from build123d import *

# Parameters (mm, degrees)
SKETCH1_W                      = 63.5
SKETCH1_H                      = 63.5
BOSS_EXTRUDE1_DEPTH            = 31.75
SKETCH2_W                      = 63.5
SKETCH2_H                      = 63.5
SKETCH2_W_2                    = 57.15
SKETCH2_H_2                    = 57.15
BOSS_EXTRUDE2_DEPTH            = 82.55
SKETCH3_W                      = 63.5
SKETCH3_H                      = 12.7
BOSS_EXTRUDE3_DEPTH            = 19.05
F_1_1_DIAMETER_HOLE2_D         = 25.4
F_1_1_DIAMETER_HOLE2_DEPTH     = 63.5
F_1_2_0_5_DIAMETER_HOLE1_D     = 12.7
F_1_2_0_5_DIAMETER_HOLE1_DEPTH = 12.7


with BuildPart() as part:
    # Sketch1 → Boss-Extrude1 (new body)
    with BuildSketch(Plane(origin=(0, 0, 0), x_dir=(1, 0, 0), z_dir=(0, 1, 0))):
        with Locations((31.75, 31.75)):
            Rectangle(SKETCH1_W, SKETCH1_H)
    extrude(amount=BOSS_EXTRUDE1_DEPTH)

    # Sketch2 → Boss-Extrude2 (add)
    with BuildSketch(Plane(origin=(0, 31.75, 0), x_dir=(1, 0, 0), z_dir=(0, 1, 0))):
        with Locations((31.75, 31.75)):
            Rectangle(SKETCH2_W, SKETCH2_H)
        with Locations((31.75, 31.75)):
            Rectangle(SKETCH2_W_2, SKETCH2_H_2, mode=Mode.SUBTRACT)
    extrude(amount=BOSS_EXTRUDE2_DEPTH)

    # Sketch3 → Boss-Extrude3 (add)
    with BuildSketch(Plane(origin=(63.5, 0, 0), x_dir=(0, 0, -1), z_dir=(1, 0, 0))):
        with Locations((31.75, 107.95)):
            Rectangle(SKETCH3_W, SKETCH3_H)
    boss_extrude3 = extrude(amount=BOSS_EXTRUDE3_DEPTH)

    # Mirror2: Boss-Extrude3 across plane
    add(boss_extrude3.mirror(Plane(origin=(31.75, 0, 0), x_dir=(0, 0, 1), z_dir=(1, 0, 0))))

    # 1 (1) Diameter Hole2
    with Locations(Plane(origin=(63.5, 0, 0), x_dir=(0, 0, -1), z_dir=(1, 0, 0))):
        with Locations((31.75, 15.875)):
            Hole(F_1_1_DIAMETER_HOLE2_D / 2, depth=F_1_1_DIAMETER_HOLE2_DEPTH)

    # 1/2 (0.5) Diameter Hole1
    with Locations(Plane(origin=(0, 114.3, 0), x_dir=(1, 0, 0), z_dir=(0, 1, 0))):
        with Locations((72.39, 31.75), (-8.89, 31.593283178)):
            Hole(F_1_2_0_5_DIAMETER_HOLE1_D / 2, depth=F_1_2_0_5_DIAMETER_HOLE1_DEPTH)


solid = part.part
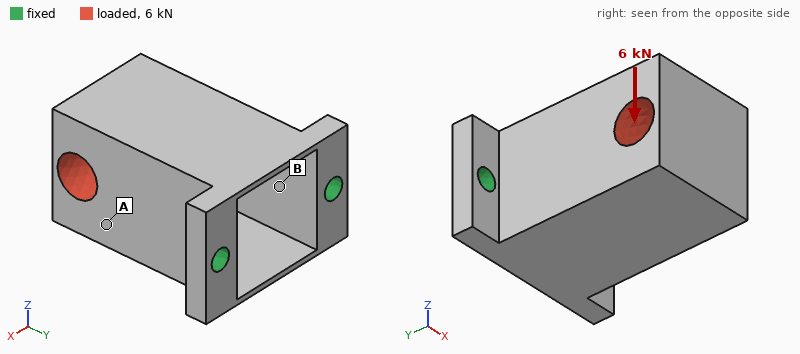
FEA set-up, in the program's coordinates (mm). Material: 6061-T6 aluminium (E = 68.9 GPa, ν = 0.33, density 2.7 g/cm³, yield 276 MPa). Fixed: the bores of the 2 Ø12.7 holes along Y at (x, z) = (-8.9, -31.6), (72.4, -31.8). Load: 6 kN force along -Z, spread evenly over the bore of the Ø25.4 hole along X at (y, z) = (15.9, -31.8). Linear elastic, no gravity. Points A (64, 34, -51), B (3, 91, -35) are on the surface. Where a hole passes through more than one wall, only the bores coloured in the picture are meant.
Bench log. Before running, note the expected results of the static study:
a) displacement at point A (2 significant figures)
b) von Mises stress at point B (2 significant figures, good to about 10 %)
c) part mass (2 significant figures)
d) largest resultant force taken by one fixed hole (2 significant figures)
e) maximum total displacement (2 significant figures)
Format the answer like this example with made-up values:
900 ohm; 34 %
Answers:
0.39 mm; 65 MPa; 500 g; 3.0 kN; 0.58 mm
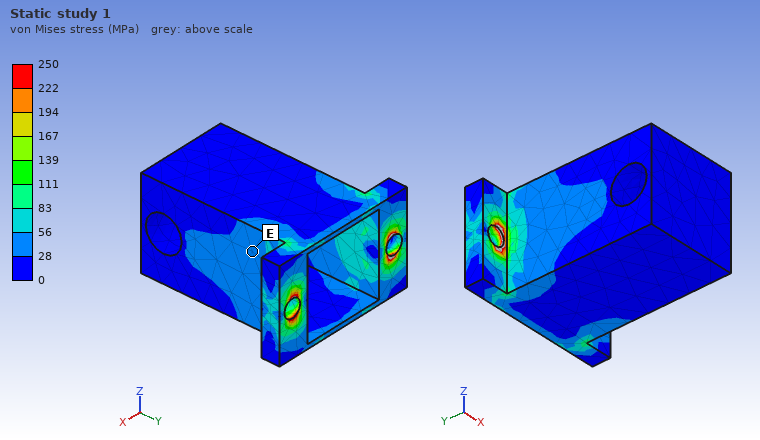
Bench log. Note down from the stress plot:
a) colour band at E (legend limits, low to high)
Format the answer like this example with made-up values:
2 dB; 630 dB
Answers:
28 to 56 MPa
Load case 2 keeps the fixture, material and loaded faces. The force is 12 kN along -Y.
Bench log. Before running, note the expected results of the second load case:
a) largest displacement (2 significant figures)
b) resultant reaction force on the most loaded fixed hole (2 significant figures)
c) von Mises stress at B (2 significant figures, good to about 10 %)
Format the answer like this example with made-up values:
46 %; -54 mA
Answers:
45 µm; 6.0 kN; 35 MPa
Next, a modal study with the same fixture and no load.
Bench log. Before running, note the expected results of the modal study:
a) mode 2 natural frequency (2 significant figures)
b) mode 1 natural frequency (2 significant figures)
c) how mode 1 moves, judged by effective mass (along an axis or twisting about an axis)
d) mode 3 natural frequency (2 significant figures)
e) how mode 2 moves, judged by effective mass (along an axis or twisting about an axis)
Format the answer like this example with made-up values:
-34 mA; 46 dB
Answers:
1700 Hz; 1000 Hz; along Z; 4000 Hz; along X
